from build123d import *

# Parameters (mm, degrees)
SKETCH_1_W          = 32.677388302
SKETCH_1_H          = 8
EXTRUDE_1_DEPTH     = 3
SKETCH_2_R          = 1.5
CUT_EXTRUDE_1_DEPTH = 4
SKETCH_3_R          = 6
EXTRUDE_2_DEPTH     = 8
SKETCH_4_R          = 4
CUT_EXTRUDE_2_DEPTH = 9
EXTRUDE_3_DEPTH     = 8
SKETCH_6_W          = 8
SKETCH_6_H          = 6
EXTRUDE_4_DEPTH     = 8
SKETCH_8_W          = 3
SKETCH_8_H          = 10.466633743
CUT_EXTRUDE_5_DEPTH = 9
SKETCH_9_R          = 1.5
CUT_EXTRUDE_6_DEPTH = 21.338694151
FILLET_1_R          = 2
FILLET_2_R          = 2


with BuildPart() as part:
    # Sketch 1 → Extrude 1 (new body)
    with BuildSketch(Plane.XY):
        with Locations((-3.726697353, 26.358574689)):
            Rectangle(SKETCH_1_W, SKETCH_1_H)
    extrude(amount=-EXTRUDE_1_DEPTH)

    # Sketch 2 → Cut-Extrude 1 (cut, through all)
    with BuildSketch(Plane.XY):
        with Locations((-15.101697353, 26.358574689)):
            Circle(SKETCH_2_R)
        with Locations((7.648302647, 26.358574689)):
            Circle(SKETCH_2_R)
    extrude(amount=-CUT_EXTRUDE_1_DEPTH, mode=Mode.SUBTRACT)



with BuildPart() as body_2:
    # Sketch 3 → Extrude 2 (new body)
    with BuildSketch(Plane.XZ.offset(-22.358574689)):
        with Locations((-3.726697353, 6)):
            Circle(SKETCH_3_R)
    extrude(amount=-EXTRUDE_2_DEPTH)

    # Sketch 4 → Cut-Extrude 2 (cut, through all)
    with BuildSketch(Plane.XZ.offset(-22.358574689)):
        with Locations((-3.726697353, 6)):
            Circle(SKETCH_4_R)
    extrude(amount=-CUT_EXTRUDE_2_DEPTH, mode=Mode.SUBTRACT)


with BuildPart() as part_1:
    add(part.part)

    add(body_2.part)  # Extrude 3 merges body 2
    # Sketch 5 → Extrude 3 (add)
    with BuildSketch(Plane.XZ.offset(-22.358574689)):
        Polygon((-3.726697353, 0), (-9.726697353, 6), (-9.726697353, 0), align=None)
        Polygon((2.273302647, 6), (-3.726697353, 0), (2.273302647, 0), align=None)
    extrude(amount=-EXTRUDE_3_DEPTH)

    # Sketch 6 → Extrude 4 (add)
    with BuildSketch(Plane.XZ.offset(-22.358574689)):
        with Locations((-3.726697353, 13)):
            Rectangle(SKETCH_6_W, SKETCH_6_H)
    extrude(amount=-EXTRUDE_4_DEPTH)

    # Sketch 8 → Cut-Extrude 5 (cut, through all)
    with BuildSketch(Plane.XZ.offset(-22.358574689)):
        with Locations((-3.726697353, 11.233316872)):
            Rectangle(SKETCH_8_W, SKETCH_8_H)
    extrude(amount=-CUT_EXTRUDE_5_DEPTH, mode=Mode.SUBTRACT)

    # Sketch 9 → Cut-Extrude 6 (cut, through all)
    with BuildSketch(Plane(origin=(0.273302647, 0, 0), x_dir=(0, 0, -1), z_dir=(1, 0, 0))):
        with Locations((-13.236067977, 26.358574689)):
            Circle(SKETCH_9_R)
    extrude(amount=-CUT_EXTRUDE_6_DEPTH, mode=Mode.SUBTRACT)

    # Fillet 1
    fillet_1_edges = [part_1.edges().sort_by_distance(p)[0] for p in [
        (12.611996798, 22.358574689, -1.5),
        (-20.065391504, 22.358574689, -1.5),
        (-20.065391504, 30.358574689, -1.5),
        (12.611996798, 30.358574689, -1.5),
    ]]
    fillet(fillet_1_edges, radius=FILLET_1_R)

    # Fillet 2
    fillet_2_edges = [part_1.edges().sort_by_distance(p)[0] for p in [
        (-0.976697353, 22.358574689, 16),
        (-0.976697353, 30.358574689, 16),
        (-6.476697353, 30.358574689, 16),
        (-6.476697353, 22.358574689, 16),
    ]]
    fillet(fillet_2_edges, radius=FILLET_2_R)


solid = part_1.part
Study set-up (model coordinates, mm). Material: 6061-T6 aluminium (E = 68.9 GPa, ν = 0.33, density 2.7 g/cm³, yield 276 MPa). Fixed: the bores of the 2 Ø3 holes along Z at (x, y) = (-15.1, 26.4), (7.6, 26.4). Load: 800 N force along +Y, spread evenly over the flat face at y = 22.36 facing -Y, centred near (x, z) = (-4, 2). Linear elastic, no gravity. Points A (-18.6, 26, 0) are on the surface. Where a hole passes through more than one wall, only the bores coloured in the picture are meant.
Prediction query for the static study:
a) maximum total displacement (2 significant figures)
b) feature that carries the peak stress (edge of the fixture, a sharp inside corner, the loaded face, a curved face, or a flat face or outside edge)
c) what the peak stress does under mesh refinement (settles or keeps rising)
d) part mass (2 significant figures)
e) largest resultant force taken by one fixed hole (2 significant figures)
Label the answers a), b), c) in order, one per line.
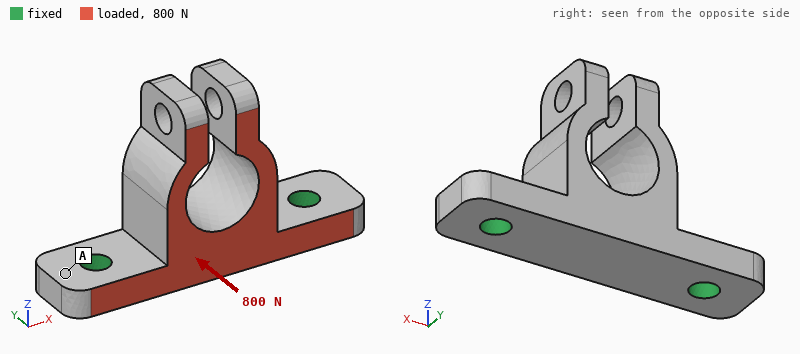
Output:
a) 100 µm
b) edge of the fixture
c) keeps rising
d) 3.9 g
e) 400 N
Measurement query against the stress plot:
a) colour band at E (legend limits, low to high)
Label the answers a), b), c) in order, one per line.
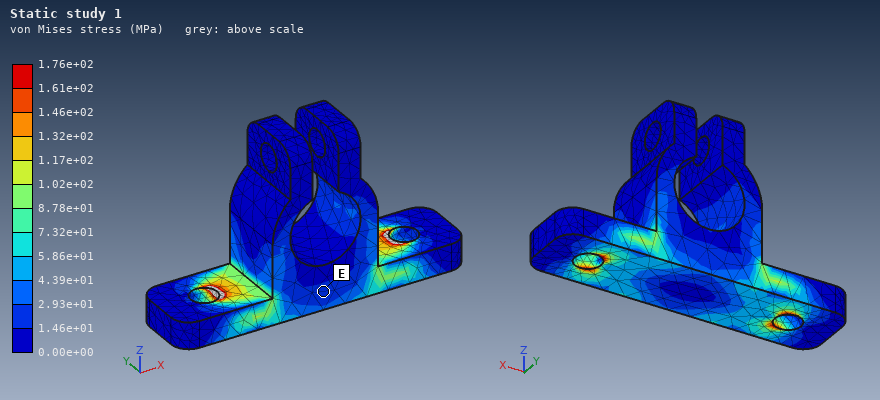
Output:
a) 1.46e+01 to 2.93e+01 MPa
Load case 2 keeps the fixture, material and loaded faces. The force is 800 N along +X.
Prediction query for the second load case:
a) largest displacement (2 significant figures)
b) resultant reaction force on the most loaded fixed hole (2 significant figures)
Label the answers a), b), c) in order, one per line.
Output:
a) 91 µm
b) 460 N
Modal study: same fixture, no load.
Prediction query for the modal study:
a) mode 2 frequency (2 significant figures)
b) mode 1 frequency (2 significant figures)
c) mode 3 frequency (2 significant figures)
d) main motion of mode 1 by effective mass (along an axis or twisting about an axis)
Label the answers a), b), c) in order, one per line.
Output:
a) 9100 Hz
b) 8700 Hz
c) 9200 Hz
d) along Y
